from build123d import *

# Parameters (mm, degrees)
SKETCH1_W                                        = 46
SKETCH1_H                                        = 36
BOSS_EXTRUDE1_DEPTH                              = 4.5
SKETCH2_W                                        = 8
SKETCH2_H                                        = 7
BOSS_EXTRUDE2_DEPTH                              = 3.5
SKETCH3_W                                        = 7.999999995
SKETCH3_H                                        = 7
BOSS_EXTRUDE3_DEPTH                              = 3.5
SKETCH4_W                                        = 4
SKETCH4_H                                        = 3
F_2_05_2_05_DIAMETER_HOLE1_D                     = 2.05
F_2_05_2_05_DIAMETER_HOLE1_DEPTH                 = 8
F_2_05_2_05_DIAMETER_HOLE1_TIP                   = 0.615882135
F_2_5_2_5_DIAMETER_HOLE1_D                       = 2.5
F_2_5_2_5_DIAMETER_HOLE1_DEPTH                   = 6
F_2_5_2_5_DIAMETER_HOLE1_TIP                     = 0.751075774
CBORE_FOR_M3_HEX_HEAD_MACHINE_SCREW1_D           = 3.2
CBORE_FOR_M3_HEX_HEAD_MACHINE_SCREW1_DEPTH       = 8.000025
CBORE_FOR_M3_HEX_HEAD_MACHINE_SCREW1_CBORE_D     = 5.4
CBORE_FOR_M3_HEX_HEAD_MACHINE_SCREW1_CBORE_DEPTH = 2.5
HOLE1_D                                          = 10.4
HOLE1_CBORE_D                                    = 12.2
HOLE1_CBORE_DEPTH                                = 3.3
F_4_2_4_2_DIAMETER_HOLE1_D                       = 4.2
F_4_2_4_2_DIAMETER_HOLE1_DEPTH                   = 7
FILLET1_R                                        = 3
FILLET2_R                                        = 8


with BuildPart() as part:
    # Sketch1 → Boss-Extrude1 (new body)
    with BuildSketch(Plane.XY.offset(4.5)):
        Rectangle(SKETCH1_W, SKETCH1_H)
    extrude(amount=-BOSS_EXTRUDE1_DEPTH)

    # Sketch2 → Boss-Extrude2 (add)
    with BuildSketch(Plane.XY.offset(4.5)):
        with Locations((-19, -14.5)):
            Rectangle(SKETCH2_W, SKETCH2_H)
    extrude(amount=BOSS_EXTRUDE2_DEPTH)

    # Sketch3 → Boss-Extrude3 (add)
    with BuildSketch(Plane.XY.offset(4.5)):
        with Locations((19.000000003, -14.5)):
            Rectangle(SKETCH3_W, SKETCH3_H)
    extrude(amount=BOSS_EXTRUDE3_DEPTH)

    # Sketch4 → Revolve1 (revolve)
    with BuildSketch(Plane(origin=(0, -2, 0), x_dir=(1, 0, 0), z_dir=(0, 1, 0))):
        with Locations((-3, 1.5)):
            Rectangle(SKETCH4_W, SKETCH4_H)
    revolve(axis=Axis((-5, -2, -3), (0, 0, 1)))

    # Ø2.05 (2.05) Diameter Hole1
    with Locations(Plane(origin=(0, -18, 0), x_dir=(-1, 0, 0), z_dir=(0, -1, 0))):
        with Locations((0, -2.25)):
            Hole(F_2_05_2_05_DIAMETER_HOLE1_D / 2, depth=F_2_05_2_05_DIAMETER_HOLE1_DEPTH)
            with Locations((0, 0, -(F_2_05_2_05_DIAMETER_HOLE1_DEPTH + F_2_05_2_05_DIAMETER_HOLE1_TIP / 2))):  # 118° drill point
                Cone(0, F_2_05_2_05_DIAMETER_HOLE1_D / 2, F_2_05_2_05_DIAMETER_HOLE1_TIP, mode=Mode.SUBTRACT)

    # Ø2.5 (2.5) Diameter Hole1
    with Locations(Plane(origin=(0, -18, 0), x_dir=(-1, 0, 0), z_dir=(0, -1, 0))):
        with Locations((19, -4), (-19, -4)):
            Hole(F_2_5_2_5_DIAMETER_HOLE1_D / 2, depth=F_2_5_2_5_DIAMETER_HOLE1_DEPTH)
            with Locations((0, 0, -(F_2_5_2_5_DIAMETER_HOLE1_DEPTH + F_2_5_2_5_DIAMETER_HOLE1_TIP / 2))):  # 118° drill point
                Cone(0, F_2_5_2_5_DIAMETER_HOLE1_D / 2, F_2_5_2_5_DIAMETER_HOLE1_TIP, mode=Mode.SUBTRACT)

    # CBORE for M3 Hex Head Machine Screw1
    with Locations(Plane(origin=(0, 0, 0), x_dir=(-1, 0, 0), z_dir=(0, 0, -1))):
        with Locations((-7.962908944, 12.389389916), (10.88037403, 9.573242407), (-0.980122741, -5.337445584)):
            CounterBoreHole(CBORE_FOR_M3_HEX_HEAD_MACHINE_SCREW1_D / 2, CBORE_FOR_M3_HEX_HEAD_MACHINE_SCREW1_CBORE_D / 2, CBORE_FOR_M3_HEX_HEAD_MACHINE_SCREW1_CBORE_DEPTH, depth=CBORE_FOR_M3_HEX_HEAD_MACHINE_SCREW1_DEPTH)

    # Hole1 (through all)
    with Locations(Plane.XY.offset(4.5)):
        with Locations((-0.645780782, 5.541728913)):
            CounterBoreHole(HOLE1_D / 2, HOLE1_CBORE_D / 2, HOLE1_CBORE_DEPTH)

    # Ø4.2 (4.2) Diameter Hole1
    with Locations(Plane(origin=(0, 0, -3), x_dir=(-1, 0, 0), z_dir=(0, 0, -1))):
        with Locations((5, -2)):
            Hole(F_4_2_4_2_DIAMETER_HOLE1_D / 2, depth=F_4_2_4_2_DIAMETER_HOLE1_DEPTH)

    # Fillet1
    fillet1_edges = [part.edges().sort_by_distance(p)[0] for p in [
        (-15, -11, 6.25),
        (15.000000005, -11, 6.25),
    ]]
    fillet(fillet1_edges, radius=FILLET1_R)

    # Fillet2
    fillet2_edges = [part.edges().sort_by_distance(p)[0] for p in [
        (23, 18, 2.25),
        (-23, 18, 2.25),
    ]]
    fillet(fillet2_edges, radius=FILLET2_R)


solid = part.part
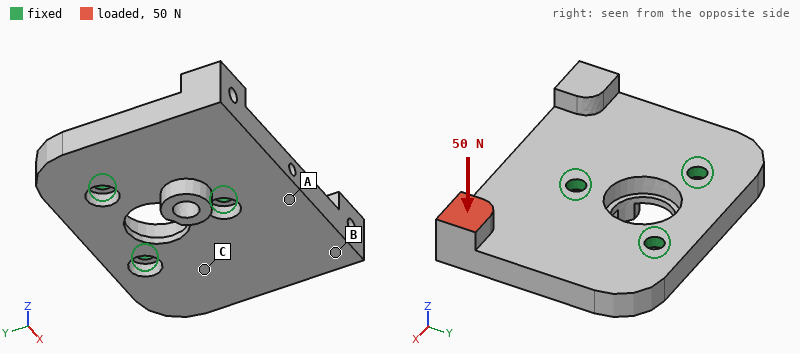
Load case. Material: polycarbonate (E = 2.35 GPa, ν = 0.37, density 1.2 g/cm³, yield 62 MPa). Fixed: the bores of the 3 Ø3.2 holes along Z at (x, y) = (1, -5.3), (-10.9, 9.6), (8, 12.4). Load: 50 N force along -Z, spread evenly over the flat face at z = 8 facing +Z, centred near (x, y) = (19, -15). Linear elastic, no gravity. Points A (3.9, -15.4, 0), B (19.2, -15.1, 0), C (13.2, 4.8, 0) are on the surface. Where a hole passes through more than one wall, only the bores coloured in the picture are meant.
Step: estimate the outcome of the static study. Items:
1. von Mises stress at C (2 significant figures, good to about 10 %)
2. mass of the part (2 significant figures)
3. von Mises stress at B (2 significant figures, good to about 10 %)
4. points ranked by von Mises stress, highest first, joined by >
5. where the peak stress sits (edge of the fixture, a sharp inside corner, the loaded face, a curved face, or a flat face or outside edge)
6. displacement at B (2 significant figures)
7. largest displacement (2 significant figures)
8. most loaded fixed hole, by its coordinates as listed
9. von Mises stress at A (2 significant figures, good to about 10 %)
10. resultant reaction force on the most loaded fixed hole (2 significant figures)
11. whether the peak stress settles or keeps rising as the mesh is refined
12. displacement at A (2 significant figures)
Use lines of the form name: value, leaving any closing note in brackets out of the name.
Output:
von Mises stress at C: 5.1 MPa
mass of the part: 8.4 g
von Mises stress at B: 2.2 MPa
points ranked by von Mises stress, highest first, joined by >: A > C > B
where the peak stress sits: edge of the fixture
displacement at B: 0.53 mm
largest displacement: 0.70 mm
most loaded fixed hole, by its coordinates as listed: (1, -5.3)
von Mises stress at A: 8.3 MPa
resultant reaction force on the most loaded fixed hole: 81 N
whether the peak stress settles or keeps rising as the mesh is refined: keeps rising
displacement at A: 0.13 mm
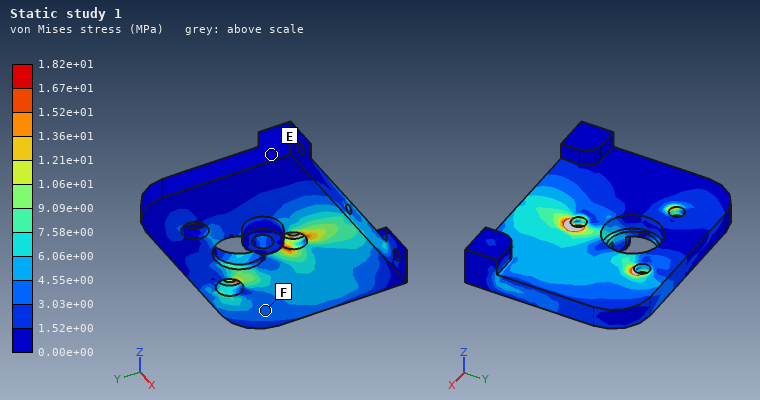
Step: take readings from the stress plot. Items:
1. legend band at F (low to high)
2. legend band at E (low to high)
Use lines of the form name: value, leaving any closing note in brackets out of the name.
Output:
legend band at F: 3.03e+00 to 4.55e+00 MPa
legend band at E: 0.00e+00 to 1.52e+00 MPa
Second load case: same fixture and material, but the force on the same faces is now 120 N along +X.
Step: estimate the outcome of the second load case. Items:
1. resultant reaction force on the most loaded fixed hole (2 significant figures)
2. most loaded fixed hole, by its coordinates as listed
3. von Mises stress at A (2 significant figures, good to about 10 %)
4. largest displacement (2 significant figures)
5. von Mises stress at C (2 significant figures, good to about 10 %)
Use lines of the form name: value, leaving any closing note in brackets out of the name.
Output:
resultant reaction force on the most loaded fixed hole: 150 N
most loaded fixed hole, by its coordinates as listed: (1, -5.3)
von Mises stress at A: 4.5 MPa
largest displacement: 0.58 mm
von Mises stress at C: 4.9 MPa
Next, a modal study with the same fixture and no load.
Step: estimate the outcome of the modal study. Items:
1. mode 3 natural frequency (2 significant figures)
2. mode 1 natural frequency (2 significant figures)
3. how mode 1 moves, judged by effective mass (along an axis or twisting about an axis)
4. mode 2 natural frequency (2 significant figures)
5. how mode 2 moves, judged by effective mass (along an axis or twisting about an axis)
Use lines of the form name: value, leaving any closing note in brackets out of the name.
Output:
mode 3 natural frequency: 3500 Hz
mode 1 natural frequency: 1400 Hz
how mode 1 moves, judged by effective mass: twisting about Y
mode 2 natural frequency: 1800 Hz
how mode 2 moves, judged by effective mass: along Z
